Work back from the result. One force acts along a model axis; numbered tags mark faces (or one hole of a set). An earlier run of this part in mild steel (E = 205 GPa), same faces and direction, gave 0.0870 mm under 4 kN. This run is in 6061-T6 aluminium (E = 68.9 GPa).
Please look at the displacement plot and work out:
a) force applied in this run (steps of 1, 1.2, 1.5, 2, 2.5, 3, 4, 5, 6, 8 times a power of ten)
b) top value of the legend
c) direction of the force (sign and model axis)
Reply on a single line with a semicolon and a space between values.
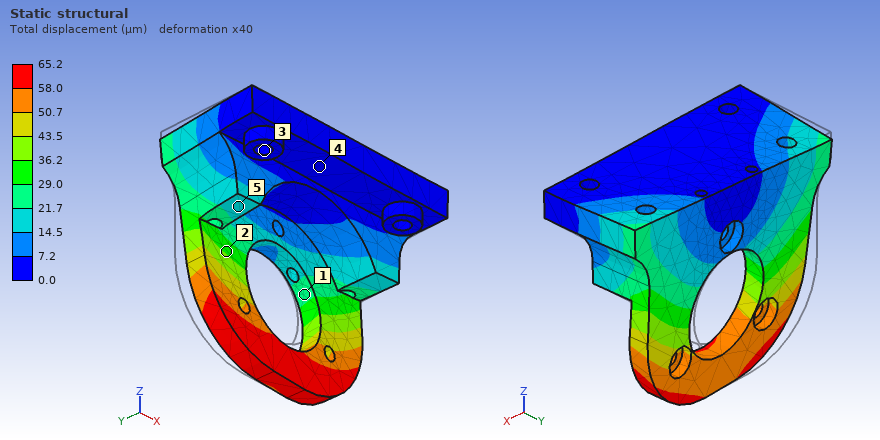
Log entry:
1 kN; 65.2 µm; +X
